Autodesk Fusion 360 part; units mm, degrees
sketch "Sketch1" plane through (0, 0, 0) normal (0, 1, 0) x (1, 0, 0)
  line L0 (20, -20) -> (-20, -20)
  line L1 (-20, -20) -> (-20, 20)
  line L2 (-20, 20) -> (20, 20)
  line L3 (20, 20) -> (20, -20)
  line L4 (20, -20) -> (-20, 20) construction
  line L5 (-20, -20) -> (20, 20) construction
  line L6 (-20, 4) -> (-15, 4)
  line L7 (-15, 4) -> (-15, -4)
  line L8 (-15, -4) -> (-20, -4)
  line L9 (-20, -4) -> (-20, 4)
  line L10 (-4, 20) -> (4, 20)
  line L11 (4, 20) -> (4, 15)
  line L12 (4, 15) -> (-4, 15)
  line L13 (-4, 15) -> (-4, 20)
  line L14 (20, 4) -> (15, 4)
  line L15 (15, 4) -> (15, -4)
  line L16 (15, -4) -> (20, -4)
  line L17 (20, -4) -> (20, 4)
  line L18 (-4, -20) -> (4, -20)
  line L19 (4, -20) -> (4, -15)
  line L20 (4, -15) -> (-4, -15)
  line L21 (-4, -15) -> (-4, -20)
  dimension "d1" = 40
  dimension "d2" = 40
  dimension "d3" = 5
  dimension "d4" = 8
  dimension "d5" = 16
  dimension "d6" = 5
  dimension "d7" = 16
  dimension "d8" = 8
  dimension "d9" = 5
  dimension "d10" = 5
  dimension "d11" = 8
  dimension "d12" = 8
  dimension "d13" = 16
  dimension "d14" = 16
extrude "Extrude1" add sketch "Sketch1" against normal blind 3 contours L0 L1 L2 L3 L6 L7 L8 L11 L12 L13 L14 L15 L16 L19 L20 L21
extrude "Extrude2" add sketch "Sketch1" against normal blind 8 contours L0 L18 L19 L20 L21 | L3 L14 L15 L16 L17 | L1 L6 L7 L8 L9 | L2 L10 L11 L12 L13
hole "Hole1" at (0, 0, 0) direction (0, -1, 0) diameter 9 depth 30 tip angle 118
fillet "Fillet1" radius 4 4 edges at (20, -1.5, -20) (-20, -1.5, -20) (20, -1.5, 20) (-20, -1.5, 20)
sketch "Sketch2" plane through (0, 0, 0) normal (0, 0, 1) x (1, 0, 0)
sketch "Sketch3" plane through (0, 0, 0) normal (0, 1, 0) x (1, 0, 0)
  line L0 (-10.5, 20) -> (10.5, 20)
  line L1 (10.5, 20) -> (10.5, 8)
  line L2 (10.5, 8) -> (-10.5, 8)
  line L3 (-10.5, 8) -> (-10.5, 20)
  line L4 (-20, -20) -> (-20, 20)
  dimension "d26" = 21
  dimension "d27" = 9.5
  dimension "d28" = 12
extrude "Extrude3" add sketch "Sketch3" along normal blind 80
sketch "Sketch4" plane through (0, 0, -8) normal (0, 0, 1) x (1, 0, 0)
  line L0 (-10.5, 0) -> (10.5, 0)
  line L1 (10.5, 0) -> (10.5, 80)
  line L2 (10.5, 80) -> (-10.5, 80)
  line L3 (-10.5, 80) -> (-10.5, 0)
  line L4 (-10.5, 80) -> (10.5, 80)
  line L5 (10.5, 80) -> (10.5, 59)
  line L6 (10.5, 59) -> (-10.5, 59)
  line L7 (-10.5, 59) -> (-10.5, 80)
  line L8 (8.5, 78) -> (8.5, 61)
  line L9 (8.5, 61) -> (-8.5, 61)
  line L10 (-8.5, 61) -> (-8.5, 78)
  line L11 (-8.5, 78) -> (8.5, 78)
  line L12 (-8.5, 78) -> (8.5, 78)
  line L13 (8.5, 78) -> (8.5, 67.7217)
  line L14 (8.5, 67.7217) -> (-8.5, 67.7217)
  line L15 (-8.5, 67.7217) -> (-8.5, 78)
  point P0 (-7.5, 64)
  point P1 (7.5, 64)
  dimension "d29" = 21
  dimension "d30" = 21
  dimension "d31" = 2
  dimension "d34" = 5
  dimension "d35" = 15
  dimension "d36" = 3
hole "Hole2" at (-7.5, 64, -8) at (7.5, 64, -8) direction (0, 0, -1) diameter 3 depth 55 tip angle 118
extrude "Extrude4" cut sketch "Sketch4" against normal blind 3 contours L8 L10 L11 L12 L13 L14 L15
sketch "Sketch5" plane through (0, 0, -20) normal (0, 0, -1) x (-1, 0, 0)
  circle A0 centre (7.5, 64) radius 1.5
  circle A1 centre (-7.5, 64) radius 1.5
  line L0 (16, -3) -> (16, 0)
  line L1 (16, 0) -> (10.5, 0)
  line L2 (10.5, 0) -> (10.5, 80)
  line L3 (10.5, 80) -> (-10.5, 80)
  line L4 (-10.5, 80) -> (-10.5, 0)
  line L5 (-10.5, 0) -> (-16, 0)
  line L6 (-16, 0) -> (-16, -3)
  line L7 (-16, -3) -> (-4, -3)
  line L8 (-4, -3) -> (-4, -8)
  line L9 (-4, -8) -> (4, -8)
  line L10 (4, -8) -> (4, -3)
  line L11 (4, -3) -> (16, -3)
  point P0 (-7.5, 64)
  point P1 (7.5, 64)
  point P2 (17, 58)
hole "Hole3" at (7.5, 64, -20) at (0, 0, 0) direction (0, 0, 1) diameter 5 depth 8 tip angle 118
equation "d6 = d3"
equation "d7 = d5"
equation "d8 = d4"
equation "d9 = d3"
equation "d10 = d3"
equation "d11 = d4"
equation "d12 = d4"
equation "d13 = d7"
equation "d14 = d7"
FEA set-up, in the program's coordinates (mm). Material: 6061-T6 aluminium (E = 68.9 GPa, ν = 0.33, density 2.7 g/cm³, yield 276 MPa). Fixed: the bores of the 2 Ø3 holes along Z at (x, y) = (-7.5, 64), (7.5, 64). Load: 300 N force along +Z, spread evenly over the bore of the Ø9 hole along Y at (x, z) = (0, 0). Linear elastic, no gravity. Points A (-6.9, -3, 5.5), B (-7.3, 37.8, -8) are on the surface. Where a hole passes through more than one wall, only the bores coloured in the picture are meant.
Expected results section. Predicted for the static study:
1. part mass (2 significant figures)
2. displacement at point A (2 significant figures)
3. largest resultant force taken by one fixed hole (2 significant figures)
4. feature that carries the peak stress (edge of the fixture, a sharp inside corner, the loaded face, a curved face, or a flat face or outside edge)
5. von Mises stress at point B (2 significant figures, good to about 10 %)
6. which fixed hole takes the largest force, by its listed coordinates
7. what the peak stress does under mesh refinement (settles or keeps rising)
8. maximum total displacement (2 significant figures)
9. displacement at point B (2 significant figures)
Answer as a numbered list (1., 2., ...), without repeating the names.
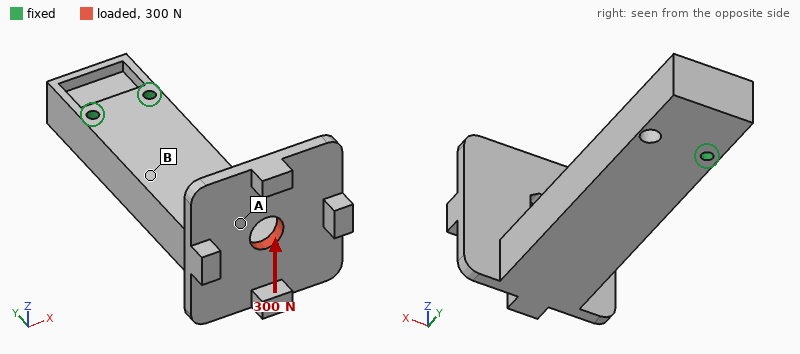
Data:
1. 67 g
2. 0.19 mm
3. 320 N
4. edge of the fixture
5. 24 MPa
6. (-7.5, 64)
7. keeps rising
8. 0.23 mm
9. 0.045 mm
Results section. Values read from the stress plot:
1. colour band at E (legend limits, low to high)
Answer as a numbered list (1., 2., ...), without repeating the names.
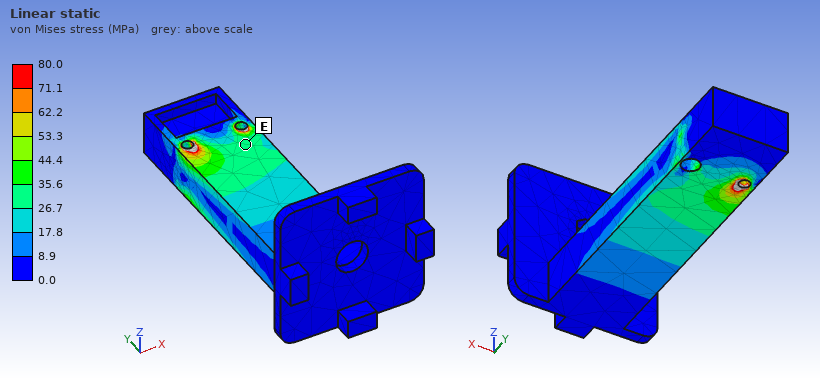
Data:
1. 26.7 to 35.6 MPa
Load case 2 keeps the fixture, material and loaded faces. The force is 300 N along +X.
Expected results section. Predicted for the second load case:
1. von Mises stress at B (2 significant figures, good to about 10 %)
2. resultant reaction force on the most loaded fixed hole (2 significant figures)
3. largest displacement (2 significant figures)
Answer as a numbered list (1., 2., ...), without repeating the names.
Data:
1. 12 MPa
2. 1.2 kN
3. 0.12 mm
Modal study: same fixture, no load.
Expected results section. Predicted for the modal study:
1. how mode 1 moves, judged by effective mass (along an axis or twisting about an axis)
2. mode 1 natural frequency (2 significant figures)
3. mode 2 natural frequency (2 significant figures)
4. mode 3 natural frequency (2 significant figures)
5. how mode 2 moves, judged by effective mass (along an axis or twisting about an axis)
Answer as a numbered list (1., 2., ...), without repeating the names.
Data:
1. along Z
2. 1200 Hz
3. 2000 Hz
4. 2400 Hz
5. along X
